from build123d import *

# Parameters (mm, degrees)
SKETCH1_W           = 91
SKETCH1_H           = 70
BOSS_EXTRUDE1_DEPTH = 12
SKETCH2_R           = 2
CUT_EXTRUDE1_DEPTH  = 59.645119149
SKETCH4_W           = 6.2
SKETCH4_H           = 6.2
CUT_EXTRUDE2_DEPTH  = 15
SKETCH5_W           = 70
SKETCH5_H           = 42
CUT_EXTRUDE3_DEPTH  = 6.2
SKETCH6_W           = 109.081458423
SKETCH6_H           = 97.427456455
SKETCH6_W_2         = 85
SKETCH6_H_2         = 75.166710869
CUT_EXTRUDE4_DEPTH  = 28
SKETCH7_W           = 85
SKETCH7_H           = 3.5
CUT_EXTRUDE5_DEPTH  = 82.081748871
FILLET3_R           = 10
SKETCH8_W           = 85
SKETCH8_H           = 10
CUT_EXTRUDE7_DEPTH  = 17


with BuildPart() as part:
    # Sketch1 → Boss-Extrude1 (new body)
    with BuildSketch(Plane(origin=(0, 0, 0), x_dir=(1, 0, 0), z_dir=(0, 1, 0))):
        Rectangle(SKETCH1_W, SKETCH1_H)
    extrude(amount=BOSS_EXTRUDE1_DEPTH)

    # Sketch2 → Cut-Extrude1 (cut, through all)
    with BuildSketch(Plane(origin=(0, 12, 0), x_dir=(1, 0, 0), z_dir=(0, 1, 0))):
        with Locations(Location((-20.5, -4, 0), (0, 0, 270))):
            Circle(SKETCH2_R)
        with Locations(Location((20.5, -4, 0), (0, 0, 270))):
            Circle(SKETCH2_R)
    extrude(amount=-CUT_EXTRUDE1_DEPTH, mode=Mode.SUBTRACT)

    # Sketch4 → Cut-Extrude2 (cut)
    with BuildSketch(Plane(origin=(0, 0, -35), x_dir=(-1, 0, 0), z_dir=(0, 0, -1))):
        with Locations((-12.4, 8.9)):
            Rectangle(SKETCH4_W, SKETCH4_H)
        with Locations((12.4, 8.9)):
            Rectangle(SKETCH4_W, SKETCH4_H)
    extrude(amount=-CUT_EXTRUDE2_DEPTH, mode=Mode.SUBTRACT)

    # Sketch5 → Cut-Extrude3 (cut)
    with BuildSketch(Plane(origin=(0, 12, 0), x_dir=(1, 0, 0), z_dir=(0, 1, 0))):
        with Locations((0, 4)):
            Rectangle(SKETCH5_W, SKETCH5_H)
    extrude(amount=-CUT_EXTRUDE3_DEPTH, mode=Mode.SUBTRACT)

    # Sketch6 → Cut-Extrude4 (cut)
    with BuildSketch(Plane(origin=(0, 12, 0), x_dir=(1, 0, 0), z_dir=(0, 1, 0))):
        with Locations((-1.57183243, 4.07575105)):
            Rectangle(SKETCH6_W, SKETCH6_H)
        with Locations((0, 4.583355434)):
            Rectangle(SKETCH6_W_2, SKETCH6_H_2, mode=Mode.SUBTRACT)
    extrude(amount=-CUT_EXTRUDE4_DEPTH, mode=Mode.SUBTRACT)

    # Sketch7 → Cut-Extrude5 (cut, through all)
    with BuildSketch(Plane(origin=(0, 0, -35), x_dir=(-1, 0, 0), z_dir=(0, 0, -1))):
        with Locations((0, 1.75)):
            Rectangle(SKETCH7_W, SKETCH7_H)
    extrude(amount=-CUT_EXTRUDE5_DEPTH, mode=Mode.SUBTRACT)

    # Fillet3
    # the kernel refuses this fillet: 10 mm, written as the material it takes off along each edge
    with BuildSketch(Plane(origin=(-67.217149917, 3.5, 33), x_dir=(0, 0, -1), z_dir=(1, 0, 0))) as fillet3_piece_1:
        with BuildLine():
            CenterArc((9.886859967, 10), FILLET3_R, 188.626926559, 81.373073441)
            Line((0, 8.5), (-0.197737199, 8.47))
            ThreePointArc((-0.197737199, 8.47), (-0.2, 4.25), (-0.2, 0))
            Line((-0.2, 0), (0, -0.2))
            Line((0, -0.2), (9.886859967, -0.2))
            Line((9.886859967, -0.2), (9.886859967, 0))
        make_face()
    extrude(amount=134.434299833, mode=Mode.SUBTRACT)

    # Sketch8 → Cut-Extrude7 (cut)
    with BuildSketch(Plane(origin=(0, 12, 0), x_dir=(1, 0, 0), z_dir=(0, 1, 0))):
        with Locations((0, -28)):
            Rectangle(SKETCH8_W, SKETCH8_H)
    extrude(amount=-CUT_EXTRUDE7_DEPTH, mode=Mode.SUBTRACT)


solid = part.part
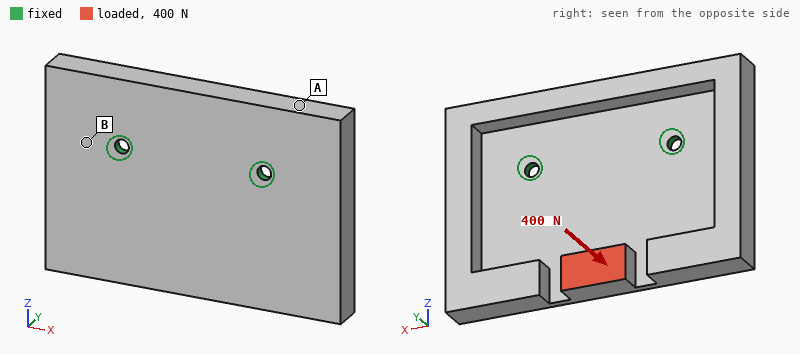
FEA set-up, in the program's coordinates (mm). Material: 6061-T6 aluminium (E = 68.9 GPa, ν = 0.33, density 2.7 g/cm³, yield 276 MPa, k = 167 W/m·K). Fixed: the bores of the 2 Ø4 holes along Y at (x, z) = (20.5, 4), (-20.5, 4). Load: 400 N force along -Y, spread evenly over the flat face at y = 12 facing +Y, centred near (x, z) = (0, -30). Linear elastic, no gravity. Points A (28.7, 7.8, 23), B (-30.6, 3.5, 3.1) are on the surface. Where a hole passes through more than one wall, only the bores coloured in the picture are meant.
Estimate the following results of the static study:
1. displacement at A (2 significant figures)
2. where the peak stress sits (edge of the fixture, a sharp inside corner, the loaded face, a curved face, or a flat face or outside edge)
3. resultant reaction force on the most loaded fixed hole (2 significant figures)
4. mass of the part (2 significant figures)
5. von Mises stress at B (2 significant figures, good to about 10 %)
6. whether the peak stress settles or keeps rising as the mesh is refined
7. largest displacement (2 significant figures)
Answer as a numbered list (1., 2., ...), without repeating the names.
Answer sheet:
1. 0.20 mm
2. edge of the fixture
3. 200 N
4. 62 g
5. 64 MPa
6. keeps rising
7. 0.68 mm
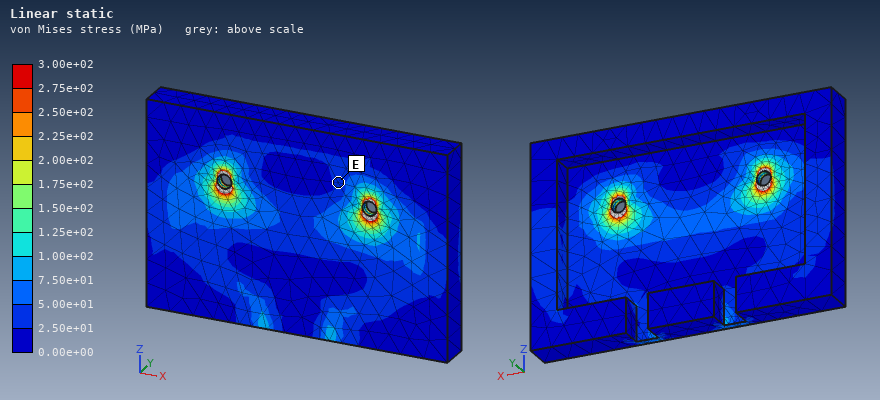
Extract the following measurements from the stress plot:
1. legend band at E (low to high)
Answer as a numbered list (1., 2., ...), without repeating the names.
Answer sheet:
1. 2.50e+01 to 5.00e+01 MPa
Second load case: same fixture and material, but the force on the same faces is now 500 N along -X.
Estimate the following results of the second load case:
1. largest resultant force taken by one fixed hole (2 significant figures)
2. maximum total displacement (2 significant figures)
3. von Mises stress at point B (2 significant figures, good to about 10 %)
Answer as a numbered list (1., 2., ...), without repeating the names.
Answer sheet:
1. 480 N
2. 89 µm
3. 14 MPa
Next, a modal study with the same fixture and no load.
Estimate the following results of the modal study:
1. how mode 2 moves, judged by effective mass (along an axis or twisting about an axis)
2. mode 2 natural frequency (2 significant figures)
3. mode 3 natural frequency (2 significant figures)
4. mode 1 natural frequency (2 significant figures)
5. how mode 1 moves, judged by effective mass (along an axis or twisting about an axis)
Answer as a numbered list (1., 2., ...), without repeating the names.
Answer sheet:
1. twisting about Z
2. 1600 Hz
3. 2600 Hz
4. 880 Hz
5. along Y
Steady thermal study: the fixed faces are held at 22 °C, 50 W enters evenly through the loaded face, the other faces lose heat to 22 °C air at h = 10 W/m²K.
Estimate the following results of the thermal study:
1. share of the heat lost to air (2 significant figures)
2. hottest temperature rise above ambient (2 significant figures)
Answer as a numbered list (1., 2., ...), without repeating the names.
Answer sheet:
1. 7.6 %
2. 86 K
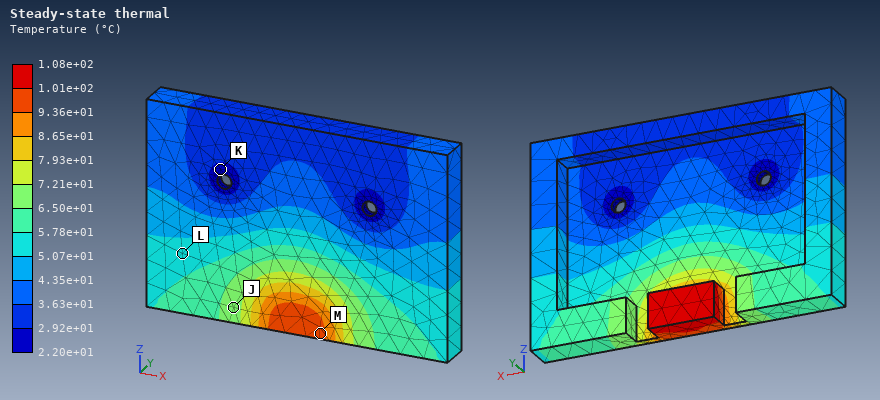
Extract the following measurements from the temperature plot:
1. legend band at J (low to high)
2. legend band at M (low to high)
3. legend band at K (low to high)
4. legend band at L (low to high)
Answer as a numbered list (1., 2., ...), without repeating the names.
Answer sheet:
1. 6.50e+01 to 7.21e+01 °C
2. 9.36e+01 to 1.01e+02 °C
3. 2.20e+01 to 2.92e+01 °C
4. 5.07e+01 to 5.78e+01 °C
